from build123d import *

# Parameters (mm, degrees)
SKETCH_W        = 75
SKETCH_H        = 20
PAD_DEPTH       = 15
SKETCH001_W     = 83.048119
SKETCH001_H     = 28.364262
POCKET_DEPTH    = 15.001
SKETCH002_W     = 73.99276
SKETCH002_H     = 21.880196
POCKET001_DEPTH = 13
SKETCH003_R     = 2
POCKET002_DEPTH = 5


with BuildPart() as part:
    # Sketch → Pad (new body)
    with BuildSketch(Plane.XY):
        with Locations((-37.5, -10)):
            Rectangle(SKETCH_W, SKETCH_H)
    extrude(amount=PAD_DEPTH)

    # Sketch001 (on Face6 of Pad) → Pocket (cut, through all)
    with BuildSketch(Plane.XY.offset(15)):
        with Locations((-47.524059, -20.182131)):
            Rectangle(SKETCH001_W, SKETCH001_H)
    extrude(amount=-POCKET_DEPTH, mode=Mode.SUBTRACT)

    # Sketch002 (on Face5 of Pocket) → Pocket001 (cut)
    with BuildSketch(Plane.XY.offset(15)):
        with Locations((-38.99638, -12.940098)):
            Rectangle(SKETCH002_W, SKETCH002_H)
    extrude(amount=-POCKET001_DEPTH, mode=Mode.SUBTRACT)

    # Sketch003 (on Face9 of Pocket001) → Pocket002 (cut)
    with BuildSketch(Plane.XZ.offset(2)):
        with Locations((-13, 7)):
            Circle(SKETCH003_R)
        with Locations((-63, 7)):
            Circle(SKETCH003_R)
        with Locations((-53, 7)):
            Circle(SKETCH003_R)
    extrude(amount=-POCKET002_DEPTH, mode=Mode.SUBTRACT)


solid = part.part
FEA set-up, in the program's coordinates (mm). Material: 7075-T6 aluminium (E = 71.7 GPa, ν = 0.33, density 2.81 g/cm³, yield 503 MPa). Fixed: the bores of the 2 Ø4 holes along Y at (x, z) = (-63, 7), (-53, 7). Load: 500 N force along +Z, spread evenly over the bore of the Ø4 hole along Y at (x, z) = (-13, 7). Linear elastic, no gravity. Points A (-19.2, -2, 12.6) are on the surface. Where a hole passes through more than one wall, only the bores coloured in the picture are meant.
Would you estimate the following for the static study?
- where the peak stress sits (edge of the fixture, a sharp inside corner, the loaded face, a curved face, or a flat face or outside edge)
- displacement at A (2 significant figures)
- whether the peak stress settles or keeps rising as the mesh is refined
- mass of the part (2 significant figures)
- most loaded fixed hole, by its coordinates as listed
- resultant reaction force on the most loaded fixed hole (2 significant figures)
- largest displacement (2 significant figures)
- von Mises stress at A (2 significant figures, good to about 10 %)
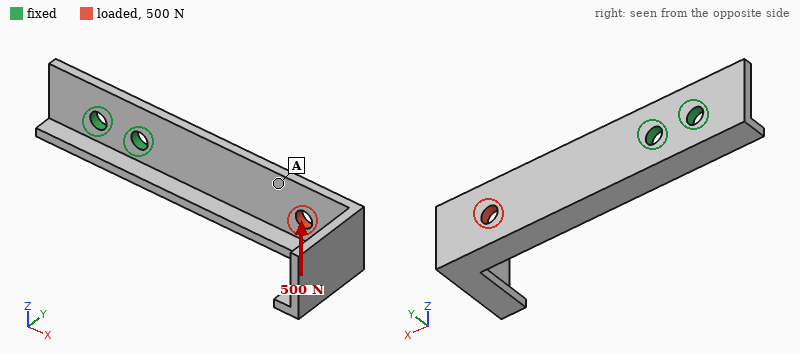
edge of the fixture
0.40 mm
keeps rising
9.6 g
(-53, 7)
1.6 kN
0.84 mm
41 MPa
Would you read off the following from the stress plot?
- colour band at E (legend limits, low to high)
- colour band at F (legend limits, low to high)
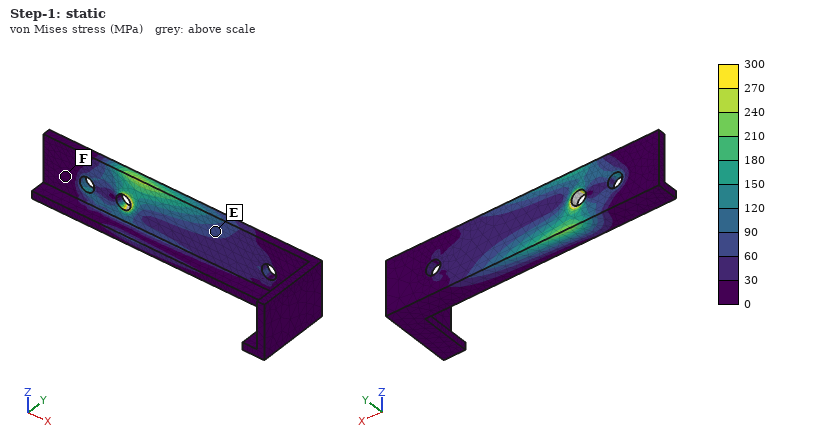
60 to 90 MPa
0 to 30 MPa
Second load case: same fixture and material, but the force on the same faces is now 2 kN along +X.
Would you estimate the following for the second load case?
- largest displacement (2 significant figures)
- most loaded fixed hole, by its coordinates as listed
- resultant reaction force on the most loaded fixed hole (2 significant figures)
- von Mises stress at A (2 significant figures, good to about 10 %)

0.32 mm
(-53, 7)
1.6 kN
44 MPa
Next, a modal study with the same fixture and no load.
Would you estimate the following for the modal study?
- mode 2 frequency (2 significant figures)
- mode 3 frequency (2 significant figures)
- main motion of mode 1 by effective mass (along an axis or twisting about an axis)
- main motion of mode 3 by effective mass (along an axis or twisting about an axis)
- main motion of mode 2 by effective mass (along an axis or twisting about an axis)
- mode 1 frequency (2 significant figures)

1300 Hz
3400 Hz
along Y
along Z
along Z
740 Hz
